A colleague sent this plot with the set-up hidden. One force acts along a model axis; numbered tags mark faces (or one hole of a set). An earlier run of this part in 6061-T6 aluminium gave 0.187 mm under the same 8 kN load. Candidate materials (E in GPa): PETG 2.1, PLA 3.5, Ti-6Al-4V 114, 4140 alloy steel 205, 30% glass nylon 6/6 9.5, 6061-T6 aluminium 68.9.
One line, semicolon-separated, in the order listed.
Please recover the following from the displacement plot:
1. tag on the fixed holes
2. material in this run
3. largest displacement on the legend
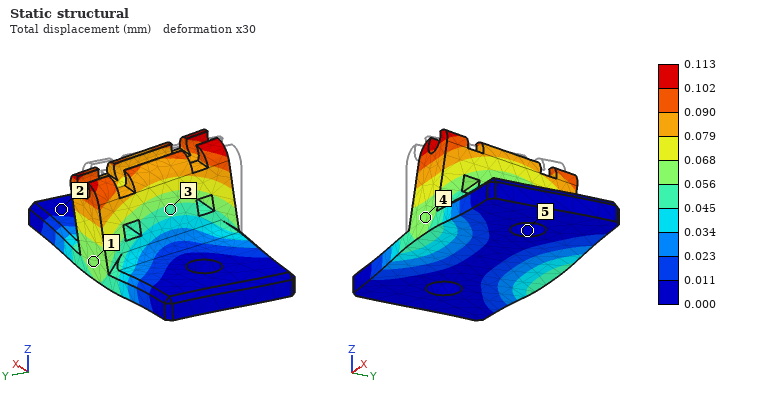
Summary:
5; Ti-6Al-4V; 0.113 mm
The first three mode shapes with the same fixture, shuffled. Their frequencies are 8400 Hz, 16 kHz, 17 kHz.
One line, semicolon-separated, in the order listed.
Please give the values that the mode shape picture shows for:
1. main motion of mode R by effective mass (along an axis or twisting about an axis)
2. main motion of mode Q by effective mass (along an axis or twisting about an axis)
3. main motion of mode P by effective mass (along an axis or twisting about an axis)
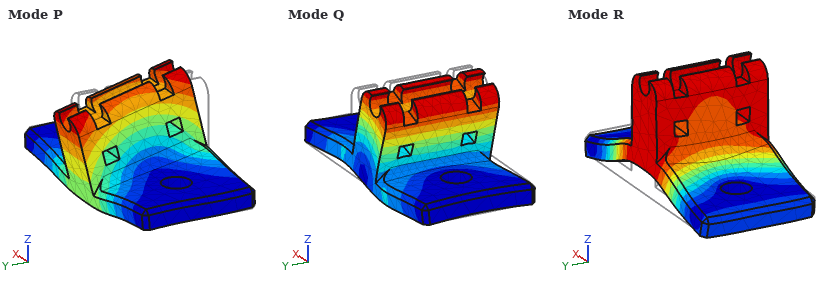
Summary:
along Z; along X; along Y
